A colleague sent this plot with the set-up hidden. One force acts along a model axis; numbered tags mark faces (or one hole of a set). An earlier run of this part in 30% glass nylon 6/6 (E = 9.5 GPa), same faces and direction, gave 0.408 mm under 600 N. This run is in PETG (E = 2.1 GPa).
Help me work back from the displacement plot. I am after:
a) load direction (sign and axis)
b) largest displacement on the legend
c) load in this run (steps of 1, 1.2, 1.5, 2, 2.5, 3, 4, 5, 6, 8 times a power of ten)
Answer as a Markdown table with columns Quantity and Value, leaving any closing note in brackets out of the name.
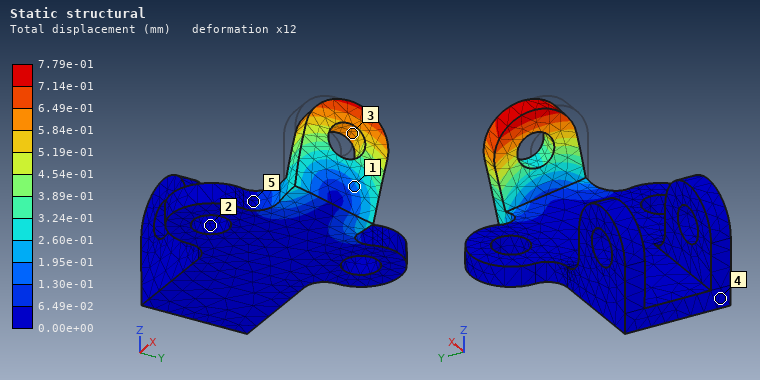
| Quantity | Value |
|---|---|
| load direction | +Y |
| largest displacement on the legend | 7.79e-01 mm |
| load in this run | 250 N |
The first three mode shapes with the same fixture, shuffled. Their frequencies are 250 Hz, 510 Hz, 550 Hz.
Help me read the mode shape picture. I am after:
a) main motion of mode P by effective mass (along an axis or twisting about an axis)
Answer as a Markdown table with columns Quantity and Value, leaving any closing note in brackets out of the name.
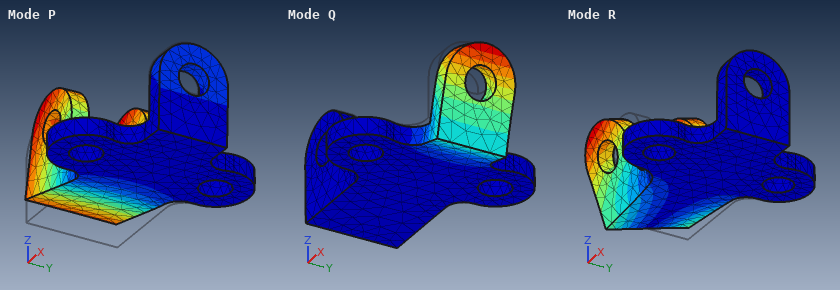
| Quantity | Value |
|---|---|
| main motion of mode P by effective mass | along Z |
